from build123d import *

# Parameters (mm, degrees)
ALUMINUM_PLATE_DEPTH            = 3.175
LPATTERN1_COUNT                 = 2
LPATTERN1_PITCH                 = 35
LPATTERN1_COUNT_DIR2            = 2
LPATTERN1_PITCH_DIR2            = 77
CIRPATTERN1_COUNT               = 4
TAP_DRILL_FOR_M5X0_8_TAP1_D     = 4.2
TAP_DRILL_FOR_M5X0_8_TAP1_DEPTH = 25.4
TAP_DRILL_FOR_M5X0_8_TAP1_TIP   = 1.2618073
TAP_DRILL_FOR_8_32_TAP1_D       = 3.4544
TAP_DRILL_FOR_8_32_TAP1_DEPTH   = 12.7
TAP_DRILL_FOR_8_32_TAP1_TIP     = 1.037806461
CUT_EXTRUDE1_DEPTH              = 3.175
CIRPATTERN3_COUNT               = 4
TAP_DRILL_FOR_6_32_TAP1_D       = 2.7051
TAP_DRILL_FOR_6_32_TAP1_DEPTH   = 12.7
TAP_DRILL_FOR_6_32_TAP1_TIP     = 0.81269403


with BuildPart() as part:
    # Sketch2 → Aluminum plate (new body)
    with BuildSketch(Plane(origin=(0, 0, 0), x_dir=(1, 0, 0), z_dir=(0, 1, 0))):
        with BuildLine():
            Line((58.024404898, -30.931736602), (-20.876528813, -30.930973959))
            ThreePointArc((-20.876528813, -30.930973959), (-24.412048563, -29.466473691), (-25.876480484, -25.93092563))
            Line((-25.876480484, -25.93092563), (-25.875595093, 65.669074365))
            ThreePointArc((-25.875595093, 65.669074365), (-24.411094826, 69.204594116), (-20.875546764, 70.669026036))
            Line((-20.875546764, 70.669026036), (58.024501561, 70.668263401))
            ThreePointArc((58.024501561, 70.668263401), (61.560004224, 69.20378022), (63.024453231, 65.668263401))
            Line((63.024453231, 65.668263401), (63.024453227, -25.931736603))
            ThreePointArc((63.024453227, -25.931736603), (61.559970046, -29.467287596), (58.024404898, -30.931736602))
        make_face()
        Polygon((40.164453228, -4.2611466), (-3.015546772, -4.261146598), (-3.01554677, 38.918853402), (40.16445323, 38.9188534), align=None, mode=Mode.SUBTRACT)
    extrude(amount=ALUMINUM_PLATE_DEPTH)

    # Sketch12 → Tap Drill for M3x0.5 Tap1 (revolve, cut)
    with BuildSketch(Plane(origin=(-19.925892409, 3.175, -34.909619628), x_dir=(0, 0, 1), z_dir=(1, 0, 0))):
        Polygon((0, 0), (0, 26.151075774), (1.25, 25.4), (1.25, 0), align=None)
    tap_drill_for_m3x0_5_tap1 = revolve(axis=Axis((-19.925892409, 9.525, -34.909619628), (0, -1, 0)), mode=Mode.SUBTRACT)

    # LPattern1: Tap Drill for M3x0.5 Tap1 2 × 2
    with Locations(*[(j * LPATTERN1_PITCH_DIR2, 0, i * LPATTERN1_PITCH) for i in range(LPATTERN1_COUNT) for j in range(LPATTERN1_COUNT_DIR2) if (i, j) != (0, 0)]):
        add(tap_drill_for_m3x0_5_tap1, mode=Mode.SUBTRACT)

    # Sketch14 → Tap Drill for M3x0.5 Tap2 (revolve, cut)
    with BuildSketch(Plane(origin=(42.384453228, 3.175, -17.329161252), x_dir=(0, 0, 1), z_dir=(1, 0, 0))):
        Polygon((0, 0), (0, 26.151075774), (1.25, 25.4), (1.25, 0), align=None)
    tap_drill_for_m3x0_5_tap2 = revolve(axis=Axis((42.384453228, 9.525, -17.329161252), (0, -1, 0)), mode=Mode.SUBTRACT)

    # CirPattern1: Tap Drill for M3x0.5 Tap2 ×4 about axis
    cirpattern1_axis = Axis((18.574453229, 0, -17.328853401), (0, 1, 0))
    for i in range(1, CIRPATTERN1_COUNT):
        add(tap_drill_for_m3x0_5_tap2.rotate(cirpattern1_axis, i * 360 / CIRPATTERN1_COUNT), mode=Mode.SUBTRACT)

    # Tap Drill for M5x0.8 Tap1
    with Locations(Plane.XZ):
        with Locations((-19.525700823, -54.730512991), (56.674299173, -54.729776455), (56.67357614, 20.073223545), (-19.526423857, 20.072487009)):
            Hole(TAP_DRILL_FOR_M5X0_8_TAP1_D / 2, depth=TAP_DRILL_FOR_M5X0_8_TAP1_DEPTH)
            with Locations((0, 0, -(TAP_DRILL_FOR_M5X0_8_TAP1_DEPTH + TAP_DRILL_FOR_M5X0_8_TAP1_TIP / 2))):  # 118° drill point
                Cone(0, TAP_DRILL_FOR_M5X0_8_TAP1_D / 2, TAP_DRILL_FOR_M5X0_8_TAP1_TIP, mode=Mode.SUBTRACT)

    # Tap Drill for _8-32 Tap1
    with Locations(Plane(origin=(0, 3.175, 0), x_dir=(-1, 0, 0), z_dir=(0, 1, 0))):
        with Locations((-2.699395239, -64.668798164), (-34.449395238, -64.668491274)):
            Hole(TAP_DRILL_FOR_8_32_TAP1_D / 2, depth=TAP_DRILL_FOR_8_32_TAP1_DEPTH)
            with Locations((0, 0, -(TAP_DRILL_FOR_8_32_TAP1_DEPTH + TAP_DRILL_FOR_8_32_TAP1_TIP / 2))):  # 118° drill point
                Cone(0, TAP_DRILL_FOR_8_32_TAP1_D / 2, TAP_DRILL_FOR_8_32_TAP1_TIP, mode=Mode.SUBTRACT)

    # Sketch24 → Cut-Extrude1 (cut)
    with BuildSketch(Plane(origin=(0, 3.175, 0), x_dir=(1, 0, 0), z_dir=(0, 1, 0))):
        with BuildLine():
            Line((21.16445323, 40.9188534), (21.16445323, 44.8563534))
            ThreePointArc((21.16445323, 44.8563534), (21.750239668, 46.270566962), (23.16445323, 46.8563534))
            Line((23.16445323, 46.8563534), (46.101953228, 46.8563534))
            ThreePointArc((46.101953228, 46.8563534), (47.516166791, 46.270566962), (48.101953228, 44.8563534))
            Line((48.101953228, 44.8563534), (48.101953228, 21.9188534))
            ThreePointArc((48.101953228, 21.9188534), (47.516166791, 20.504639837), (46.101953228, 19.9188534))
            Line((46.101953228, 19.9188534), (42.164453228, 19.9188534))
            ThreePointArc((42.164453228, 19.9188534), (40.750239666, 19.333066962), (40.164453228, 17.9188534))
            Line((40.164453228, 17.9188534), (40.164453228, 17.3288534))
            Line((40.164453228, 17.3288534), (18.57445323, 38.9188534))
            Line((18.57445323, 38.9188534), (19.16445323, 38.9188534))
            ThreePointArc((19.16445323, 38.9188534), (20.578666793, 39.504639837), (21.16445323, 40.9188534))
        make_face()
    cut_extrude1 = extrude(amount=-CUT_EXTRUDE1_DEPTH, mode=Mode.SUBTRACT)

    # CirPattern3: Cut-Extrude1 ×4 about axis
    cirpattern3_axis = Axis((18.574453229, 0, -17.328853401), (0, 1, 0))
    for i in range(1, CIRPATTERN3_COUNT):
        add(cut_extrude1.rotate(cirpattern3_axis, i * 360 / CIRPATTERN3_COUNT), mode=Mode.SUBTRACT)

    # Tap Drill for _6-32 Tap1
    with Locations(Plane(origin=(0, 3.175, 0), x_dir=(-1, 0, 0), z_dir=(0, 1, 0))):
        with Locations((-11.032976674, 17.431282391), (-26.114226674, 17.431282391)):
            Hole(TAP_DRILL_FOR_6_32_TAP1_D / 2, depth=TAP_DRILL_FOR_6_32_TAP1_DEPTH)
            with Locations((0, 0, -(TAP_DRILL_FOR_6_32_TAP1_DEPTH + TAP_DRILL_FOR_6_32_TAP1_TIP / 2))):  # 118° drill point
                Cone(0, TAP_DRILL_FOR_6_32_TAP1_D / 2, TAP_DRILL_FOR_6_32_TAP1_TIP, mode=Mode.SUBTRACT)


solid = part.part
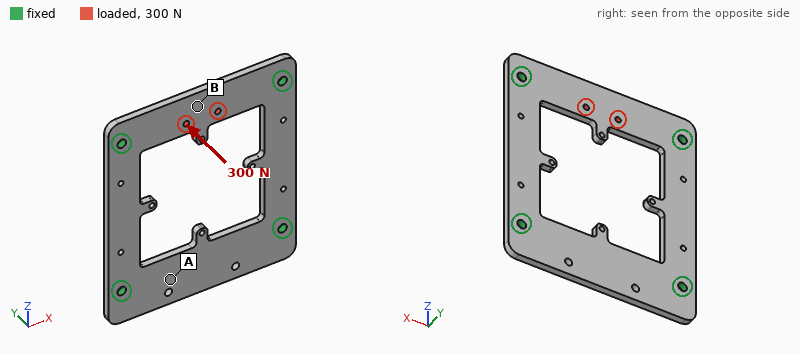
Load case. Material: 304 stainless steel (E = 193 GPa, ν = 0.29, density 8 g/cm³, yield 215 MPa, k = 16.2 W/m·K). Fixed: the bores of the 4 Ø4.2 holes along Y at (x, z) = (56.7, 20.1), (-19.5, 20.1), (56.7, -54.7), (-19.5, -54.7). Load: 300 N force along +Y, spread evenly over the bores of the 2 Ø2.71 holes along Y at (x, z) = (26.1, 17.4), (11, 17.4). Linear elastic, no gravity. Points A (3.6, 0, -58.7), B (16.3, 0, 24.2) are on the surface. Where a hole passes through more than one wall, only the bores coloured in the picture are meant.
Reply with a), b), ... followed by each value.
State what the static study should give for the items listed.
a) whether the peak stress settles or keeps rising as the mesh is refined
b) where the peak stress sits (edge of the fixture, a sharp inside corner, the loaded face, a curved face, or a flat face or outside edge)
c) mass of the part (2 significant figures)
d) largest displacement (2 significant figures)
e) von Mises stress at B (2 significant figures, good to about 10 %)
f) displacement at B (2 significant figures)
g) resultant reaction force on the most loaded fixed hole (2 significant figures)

a) keeps rising
b) edge of the fixture
c) 140 g
d) 81 µm
e) 52 MPa
f) 56 µm
g) 150 N
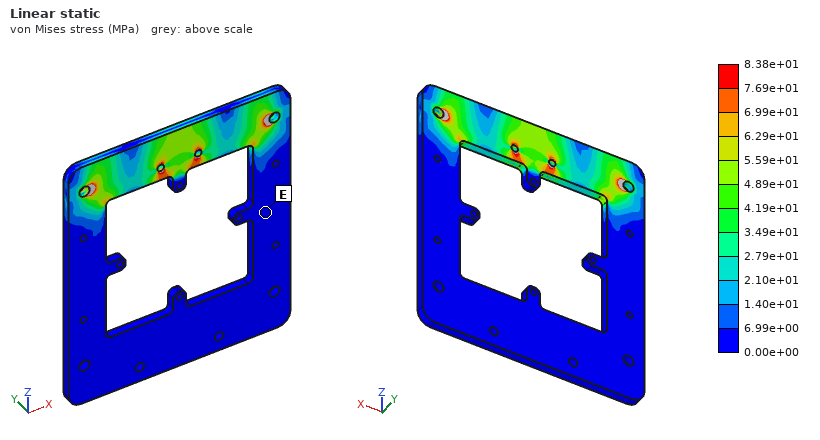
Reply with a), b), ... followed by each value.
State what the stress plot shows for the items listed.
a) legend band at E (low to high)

a) 0.00e+00 to 6.99e+00 MPa
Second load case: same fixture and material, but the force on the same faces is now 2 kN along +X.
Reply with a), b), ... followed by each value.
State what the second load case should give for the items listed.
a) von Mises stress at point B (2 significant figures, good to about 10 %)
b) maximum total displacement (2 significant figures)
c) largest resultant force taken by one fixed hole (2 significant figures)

a) 7.0 MPa
b) 4.8 µm
c) 1.0 kN
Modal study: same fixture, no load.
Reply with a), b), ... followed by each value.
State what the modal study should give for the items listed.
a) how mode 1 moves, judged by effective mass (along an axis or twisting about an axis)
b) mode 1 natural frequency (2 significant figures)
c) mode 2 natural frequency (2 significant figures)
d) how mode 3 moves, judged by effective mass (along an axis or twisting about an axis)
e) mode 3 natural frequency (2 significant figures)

a) along Y
b) 2600 Hz
c) 2800 Hz
d) along Y
e) 2900 Hz
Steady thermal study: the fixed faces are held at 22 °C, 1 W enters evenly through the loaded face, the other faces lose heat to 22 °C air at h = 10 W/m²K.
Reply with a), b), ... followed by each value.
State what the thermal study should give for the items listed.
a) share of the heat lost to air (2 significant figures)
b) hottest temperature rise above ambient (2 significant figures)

a) 29 %
b) 15 K
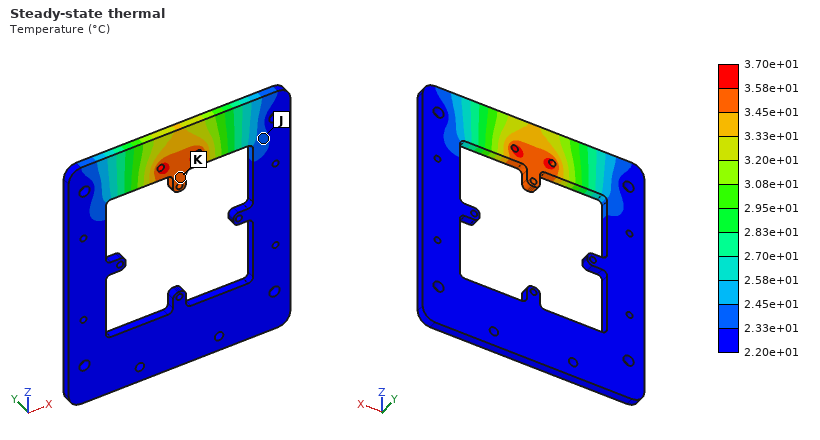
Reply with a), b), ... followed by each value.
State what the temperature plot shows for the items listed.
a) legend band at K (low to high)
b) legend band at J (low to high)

a) 3.45e+01 to 3.58e+01 °C
b) 2.33e+01 to 2.45e+01 °C
